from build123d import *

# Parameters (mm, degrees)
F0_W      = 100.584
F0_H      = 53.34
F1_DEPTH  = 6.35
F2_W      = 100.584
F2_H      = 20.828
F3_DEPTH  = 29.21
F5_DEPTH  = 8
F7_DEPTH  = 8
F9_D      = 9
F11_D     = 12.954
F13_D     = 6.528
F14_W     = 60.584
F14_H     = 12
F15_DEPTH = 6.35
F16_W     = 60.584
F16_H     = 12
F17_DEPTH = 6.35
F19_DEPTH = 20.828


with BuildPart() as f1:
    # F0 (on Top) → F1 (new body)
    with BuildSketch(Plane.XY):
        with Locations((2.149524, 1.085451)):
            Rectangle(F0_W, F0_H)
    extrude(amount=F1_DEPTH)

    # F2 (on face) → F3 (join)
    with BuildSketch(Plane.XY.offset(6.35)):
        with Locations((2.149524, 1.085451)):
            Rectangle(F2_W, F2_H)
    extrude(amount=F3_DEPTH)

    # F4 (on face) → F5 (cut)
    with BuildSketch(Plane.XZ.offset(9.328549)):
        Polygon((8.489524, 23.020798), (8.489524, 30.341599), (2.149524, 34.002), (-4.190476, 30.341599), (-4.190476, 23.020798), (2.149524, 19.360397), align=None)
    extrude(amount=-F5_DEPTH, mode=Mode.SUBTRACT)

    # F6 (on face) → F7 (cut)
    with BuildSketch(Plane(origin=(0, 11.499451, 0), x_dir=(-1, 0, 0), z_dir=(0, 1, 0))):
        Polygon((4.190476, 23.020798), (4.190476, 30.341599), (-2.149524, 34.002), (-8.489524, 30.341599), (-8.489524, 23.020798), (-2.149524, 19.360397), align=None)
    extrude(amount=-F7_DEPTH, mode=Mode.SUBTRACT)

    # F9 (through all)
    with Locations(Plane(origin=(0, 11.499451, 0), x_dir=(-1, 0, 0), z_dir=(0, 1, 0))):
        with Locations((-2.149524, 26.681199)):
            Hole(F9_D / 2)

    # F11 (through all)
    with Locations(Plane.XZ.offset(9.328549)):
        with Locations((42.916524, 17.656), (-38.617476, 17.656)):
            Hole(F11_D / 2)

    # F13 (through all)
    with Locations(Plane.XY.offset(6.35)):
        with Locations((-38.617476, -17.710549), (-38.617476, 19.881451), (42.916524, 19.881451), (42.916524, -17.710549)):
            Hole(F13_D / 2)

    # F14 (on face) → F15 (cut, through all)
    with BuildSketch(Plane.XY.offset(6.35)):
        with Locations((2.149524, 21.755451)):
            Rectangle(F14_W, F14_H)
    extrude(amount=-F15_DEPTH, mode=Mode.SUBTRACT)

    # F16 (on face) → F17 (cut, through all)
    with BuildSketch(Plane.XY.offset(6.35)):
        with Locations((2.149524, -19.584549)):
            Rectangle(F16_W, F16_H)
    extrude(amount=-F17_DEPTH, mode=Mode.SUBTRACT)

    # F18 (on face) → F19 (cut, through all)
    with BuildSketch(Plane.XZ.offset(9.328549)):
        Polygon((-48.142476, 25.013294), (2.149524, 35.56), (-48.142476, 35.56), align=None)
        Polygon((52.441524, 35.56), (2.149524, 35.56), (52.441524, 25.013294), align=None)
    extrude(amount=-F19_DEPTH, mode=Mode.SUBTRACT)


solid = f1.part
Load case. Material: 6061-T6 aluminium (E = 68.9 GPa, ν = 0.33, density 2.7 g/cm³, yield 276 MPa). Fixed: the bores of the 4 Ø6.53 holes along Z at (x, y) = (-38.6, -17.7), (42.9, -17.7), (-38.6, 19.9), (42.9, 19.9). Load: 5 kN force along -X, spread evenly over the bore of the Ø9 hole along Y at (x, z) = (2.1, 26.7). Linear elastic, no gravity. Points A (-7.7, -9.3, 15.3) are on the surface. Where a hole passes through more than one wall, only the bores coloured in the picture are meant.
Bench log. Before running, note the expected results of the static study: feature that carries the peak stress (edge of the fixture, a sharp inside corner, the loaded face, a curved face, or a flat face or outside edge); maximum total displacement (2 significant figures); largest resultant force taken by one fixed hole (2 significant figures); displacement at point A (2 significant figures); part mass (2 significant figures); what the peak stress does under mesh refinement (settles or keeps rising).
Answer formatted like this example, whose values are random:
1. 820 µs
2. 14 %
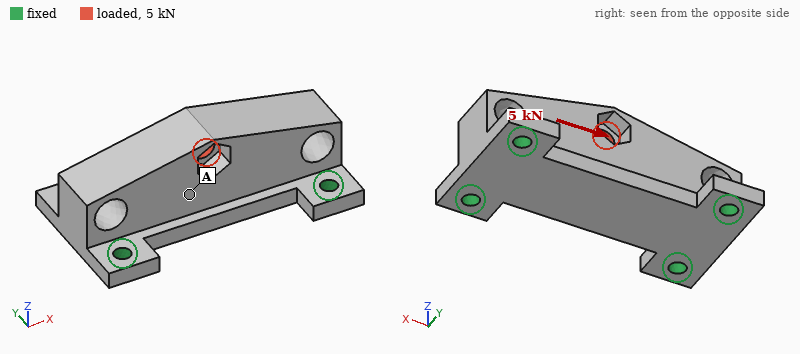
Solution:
1. edge of the fixture
2. 17 µm
3. 1.6 kN
4. 7.4 µm
5. 180 g
6. keeps rising
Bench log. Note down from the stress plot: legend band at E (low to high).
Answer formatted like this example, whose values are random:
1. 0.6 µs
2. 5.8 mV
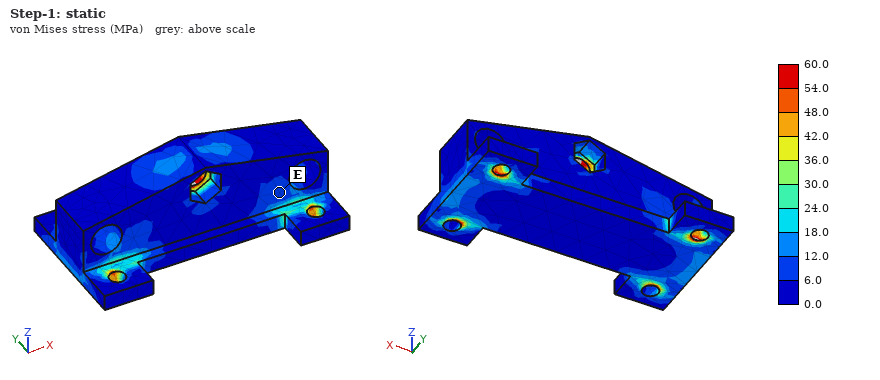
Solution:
1. 6.0 to 12.0 MPa
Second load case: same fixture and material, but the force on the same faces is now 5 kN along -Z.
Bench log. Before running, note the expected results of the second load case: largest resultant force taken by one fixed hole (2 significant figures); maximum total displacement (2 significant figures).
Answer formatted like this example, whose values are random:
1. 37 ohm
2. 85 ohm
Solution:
1. 1.6 kN
2. 29 µm
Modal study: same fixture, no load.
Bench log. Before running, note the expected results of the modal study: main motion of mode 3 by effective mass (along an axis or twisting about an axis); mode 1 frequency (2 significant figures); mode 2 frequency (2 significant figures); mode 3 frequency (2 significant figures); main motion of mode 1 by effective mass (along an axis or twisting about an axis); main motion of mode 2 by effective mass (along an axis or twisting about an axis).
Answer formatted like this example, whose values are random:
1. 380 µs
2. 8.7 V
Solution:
1. along X
2. 6600 Hz
3. 7300 Hz
4. 11 kHz
5. along Y
6. along Z
